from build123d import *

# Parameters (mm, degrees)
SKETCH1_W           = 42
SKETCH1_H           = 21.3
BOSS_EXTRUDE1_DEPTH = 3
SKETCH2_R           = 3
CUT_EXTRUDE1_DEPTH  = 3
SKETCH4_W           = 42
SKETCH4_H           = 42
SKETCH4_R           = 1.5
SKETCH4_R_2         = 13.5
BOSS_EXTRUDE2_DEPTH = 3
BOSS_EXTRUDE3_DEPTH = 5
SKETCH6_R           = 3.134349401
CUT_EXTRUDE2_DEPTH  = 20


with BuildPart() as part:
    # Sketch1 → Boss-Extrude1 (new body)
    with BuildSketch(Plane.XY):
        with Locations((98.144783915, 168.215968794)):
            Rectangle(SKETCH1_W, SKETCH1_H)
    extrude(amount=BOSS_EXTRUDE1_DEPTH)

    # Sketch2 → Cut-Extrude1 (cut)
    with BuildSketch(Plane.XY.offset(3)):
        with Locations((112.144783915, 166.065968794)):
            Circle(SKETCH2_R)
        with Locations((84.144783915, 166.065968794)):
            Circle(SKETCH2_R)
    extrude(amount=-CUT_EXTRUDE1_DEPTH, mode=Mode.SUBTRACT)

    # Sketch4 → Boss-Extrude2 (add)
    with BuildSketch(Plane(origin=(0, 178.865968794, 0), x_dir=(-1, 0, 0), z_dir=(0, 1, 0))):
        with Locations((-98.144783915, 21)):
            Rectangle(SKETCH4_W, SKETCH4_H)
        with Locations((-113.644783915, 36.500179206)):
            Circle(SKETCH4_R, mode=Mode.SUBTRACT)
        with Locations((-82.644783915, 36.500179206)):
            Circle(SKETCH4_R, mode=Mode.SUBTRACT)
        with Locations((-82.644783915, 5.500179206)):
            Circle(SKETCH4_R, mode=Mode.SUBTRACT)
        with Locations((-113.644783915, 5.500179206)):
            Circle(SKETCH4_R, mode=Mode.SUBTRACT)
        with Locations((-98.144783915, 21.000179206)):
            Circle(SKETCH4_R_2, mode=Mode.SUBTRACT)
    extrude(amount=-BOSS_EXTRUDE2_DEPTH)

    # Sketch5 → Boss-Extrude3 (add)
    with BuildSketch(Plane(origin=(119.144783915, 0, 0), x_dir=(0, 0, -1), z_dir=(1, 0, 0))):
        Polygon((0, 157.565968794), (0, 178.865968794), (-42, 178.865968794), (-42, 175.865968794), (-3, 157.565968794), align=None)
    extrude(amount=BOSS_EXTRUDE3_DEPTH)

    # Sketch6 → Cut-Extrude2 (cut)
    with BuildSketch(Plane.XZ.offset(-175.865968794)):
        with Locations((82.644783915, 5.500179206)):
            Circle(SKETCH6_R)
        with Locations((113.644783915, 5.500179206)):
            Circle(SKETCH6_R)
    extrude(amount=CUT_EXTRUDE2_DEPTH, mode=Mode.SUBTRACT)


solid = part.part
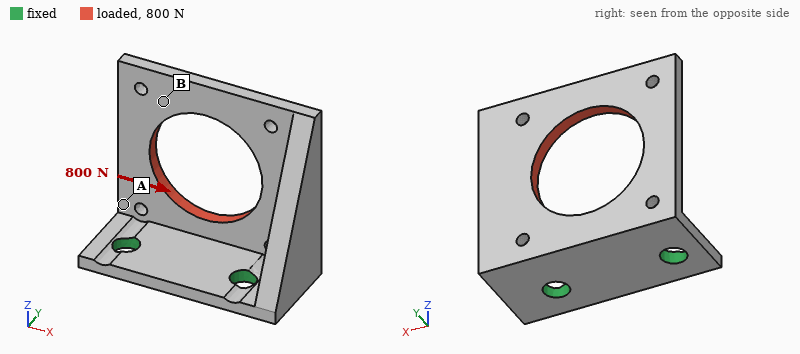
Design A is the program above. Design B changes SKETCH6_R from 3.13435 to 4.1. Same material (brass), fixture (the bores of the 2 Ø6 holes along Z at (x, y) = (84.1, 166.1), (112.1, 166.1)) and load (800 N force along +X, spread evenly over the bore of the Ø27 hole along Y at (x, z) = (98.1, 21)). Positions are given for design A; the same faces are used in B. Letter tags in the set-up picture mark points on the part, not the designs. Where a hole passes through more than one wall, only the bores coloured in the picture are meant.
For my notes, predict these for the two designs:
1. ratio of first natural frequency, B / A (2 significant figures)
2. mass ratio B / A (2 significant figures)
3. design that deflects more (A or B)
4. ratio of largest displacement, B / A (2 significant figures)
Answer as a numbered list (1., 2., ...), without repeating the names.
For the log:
1. 0.88
2. 0.98
3. B
4. 1.5
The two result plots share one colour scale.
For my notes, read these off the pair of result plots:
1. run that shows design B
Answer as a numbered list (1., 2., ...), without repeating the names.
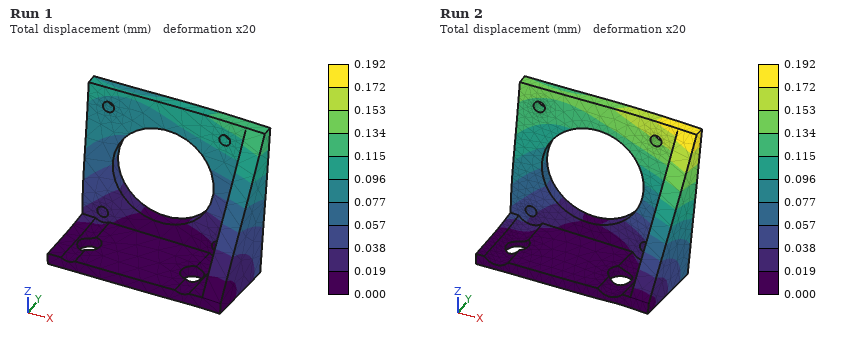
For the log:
1. Run 2
